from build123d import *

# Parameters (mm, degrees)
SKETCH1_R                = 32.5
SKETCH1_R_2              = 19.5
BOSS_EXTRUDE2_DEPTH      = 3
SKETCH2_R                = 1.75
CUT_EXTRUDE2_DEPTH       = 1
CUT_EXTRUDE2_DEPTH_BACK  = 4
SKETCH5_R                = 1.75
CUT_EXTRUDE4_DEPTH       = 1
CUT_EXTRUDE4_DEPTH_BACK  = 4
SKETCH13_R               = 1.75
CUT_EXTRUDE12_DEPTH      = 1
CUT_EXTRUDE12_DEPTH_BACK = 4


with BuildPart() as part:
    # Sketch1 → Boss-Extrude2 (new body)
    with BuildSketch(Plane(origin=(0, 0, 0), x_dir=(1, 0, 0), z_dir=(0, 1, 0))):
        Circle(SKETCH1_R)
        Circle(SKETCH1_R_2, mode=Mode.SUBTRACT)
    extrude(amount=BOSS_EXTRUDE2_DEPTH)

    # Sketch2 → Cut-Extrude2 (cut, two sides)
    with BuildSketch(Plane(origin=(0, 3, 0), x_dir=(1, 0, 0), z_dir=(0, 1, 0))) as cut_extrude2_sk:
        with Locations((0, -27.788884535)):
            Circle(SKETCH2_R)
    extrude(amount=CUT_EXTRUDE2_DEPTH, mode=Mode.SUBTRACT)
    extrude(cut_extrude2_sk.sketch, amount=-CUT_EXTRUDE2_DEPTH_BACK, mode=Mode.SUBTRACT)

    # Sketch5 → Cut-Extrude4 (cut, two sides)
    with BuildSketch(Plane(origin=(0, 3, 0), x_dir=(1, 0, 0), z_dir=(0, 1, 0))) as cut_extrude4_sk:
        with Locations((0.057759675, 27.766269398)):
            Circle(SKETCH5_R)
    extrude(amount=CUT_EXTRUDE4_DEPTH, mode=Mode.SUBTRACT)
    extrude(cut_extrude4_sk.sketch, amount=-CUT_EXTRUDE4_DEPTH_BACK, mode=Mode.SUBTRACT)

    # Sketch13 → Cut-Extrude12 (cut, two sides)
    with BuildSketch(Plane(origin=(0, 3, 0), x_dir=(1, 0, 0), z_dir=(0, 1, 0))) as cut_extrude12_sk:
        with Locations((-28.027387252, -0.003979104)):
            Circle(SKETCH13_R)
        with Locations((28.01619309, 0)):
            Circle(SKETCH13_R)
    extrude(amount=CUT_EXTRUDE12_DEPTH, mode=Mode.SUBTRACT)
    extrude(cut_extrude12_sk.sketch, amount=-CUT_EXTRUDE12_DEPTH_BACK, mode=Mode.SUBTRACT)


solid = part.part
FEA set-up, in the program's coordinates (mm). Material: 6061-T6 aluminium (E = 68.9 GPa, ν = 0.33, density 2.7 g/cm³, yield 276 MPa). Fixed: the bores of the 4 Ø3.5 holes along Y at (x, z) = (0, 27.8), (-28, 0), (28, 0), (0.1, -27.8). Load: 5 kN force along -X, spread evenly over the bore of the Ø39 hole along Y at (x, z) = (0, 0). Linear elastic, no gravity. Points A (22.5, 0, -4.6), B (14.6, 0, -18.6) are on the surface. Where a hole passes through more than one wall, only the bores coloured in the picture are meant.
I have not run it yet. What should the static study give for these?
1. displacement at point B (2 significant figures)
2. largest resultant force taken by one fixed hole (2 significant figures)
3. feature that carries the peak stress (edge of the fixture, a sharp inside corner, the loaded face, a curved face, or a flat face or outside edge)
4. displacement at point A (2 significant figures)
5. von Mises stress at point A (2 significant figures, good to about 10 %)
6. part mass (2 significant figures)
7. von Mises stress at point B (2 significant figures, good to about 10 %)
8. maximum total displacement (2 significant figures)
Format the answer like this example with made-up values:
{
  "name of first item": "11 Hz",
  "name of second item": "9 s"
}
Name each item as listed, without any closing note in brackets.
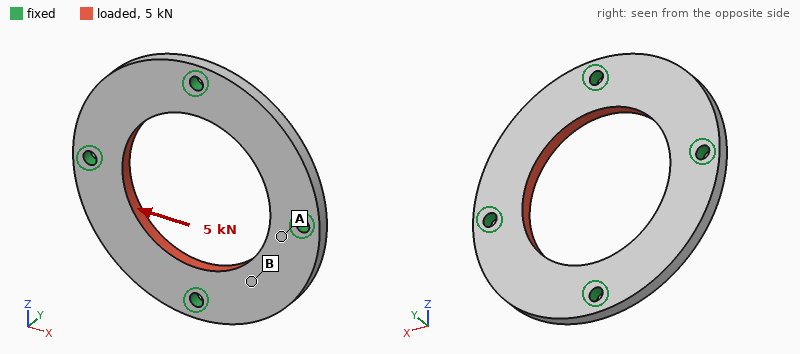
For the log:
{
  "displacement at point B": "9.7 µm",
  "largest resultant force taken by one fixed hole": "1.5 kN",
  "feature that carries the peak stress": "edge of the fixture",
  "displacement at point A": "4.0 µm",
  "von Mises stress at point A": "31 MPa",
  "part mass": "17 g",
  "von Mises stress at point B": "12 MPa",
  "maximum total displacement": "11 µm"
}
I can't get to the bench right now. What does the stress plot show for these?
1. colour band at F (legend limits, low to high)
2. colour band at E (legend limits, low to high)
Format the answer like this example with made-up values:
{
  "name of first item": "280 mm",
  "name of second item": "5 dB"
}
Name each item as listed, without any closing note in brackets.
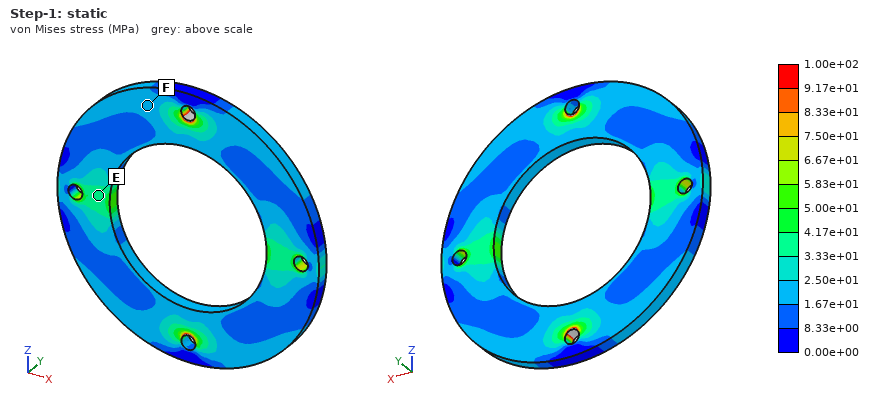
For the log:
{
  "colour band at F": "1.67e+01 to 2.50e+01 MPa",
  "colour band at E": "3.33e+01 to 4.17e+01 MPa"
}
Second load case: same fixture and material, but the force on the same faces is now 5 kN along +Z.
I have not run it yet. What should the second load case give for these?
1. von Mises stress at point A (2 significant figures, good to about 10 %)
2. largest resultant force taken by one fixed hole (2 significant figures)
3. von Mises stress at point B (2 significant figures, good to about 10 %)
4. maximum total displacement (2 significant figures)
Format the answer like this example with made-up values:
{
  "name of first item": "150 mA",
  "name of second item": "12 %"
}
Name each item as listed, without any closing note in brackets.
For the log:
{
  "von Mises stress at point A": "24 MPa",
  "largest resultant force taken by one fixed hole": "1.5 kN",
  "von Mises stress at point B": "14 MPa",
  "maximum total displacement": "11 µm"
}
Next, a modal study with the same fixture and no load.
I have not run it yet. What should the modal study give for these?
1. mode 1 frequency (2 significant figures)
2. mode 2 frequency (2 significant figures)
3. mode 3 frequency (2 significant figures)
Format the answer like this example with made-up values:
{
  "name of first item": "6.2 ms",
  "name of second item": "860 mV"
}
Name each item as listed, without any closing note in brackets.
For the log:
{
  "mode 1 frequency": "7800 Hz",
  "mode 2 frequency": "8200 Hz",
  "mode 3 frequency": "8200 Hz"
}
